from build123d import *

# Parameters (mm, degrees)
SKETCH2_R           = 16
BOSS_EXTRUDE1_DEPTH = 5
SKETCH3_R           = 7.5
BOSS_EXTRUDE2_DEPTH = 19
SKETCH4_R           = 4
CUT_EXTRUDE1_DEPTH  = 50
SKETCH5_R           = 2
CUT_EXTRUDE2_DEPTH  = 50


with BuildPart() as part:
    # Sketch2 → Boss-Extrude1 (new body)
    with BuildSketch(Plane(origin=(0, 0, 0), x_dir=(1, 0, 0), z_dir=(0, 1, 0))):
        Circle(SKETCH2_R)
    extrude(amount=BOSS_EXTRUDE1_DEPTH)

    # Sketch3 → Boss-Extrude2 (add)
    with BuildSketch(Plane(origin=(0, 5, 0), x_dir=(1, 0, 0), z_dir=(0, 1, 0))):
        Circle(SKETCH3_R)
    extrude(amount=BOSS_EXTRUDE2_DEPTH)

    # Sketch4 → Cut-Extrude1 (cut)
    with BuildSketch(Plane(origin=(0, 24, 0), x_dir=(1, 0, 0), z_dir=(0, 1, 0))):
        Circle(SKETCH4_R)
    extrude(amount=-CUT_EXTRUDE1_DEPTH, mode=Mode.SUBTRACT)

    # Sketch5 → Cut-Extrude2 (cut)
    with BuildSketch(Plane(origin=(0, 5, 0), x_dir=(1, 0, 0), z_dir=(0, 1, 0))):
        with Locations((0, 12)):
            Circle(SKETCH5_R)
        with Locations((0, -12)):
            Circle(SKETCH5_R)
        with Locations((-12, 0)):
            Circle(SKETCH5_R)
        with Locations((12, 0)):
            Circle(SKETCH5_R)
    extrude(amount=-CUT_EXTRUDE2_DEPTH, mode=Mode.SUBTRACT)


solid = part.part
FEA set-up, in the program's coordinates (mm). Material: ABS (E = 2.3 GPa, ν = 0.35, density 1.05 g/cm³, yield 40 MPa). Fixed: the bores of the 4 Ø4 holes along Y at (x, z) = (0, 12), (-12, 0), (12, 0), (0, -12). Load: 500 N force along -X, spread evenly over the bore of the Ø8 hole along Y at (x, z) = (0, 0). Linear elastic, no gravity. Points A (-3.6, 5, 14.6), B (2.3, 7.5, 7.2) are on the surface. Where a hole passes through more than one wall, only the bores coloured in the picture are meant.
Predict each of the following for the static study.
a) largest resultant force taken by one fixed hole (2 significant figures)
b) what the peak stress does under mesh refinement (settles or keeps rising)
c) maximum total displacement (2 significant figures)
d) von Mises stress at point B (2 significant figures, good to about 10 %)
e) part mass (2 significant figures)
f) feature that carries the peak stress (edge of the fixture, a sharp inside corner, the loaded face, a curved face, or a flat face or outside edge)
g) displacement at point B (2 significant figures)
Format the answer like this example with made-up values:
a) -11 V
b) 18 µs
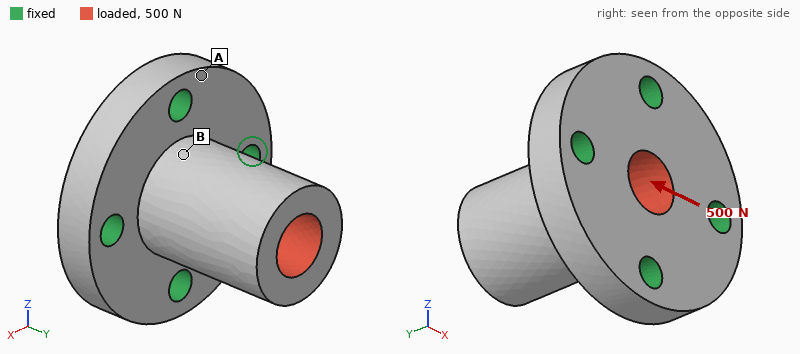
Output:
a) 280 N
b) keeps rising
c) 0.23 mm
d) 5.3 MPa
e) 6.2 g
f) edge of the fixture
g) 0.040 mm
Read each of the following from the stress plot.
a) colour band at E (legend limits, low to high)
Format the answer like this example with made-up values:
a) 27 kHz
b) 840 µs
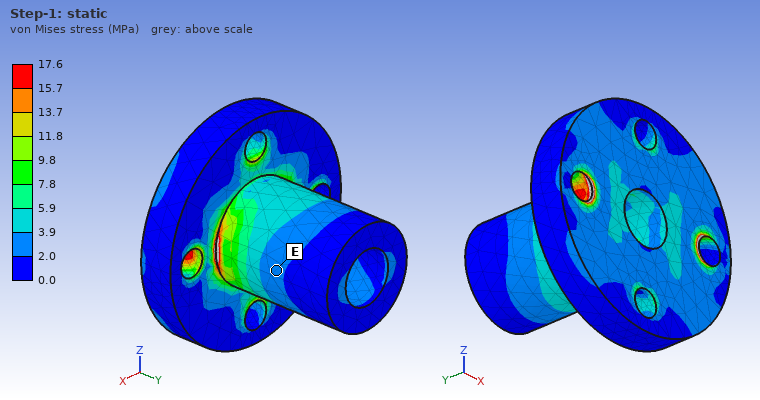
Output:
a) 2.0 to 3.9 MPa
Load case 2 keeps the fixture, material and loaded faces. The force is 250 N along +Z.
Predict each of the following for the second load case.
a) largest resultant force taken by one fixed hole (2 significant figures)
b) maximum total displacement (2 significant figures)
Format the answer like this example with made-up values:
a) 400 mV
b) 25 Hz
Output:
a) 140 N
b) 0.12 mm
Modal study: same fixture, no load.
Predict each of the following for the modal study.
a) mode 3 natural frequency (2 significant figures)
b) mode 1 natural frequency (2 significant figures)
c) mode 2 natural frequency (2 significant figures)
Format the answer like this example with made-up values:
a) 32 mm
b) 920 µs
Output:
a) 11 kHz
b) 4900 Hz
c) 4900 Hz
